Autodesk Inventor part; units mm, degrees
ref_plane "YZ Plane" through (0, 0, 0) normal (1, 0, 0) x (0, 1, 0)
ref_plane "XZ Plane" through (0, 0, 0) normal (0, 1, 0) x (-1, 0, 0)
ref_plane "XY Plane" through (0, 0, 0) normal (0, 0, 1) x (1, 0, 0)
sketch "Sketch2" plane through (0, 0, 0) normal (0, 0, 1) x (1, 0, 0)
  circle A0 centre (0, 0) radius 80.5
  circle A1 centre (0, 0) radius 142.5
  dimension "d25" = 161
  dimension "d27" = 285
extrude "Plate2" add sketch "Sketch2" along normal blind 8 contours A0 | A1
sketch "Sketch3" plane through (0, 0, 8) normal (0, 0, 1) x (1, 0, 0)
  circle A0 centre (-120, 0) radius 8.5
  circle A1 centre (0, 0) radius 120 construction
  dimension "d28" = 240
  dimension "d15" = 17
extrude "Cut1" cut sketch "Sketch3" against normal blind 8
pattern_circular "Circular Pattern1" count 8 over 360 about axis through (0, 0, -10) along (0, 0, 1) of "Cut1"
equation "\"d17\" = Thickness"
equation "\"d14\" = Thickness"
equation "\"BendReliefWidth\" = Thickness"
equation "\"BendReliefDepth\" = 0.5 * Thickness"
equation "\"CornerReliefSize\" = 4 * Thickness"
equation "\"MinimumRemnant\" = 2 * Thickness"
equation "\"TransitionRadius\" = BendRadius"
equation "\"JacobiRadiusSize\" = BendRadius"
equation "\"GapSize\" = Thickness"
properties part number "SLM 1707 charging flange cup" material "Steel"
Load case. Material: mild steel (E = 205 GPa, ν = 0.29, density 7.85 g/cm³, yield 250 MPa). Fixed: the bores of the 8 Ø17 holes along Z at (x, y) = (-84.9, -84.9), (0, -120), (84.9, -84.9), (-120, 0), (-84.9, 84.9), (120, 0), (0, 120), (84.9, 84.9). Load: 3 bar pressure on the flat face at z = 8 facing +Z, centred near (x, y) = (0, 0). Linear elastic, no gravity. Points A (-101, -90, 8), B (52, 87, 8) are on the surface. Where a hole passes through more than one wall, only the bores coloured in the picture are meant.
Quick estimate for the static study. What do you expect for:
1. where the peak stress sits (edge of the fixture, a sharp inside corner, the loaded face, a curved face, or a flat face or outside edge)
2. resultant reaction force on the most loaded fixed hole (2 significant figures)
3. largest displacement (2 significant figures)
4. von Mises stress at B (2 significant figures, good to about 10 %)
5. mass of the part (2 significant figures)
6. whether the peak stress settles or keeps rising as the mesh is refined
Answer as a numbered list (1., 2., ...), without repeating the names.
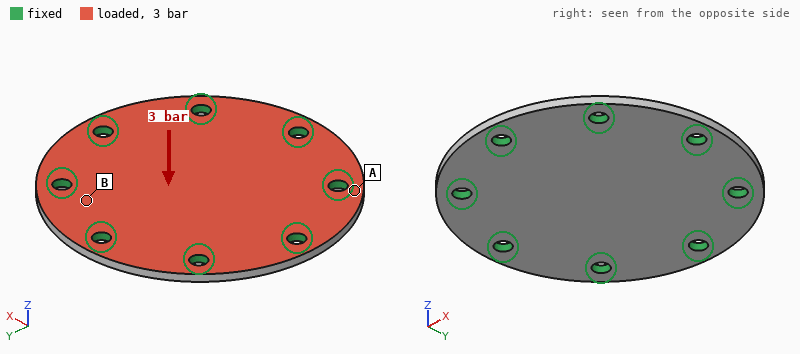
1. edge of the fixture
2. 2.3 kN
3. 0.10 mm
4. 26 MPa
5. 3.9 kg
6. keeps rising
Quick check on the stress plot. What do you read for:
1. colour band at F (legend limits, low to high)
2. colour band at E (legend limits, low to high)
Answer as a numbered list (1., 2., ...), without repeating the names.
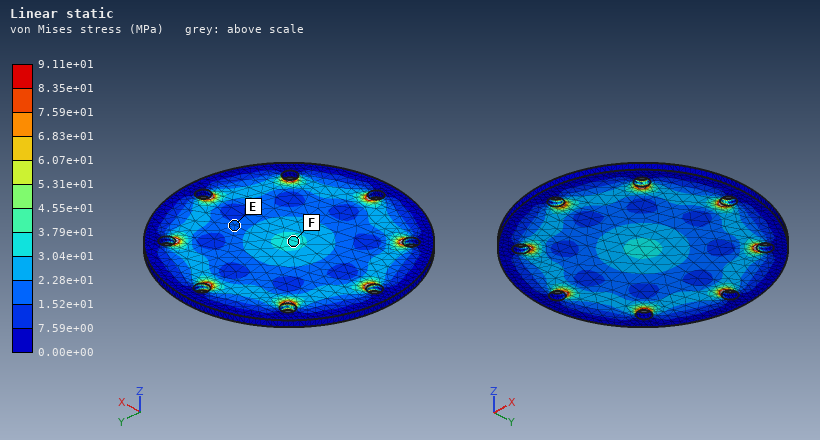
1. 3.04e+01 to 3.79e+01 MPa
2. 1.52e+01 to 2.28e+01 MPa
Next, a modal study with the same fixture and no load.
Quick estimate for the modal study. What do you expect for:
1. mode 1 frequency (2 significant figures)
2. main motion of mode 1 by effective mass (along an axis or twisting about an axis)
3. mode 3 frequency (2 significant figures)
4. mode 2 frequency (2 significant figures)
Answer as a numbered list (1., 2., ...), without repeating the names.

1. 1400 Hz
2. along Z
3. 2800 Hz
4. 2800 Hz
